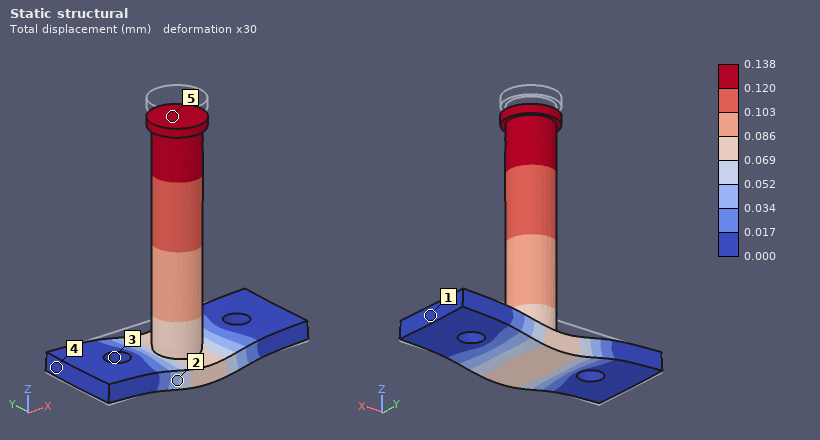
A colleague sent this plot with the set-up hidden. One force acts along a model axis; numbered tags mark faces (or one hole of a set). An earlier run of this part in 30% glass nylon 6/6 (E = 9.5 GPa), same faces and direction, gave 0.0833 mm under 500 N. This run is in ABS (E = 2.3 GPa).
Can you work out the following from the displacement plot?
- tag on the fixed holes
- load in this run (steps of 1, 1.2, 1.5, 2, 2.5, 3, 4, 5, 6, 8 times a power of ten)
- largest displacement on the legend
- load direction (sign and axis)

3
200 N
0.138 mm
-Z
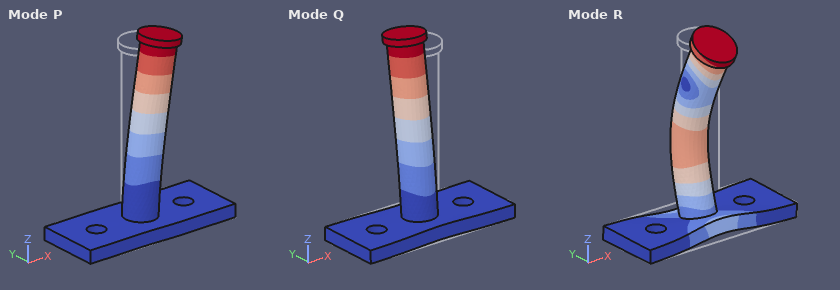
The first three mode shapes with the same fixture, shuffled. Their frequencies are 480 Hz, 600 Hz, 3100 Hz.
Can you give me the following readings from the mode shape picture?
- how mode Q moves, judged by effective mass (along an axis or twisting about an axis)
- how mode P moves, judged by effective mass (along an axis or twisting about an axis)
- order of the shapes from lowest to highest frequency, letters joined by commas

along Y
along X
Q, P, R
